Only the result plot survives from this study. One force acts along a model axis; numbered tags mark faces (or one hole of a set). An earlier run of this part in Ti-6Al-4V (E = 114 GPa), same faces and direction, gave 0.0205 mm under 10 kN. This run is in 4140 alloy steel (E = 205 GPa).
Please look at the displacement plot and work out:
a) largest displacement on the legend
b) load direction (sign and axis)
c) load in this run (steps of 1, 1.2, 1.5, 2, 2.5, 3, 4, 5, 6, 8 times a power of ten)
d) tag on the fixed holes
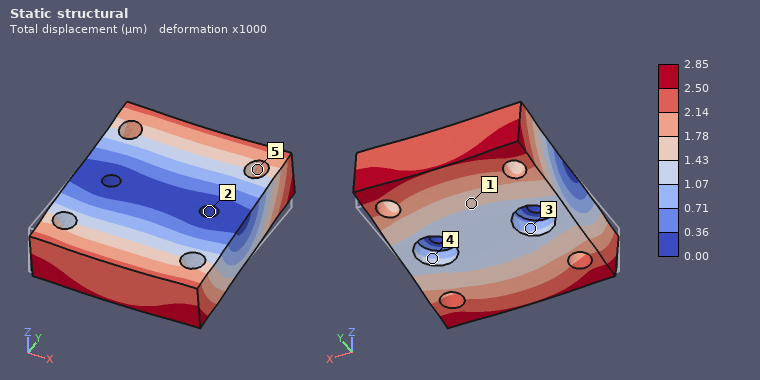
2.85 µm
+Y
2.5 kN
2
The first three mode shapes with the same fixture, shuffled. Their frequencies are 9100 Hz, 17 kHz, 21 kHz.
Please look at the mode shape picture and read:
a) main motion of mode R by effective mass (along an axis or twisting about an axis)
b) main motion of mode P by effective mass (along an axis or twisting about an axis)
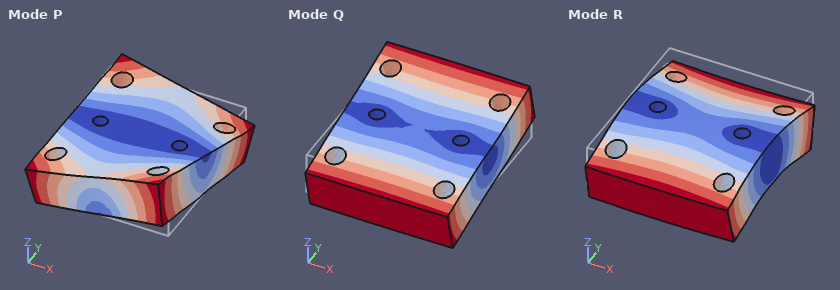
along Z
twisting about Z
